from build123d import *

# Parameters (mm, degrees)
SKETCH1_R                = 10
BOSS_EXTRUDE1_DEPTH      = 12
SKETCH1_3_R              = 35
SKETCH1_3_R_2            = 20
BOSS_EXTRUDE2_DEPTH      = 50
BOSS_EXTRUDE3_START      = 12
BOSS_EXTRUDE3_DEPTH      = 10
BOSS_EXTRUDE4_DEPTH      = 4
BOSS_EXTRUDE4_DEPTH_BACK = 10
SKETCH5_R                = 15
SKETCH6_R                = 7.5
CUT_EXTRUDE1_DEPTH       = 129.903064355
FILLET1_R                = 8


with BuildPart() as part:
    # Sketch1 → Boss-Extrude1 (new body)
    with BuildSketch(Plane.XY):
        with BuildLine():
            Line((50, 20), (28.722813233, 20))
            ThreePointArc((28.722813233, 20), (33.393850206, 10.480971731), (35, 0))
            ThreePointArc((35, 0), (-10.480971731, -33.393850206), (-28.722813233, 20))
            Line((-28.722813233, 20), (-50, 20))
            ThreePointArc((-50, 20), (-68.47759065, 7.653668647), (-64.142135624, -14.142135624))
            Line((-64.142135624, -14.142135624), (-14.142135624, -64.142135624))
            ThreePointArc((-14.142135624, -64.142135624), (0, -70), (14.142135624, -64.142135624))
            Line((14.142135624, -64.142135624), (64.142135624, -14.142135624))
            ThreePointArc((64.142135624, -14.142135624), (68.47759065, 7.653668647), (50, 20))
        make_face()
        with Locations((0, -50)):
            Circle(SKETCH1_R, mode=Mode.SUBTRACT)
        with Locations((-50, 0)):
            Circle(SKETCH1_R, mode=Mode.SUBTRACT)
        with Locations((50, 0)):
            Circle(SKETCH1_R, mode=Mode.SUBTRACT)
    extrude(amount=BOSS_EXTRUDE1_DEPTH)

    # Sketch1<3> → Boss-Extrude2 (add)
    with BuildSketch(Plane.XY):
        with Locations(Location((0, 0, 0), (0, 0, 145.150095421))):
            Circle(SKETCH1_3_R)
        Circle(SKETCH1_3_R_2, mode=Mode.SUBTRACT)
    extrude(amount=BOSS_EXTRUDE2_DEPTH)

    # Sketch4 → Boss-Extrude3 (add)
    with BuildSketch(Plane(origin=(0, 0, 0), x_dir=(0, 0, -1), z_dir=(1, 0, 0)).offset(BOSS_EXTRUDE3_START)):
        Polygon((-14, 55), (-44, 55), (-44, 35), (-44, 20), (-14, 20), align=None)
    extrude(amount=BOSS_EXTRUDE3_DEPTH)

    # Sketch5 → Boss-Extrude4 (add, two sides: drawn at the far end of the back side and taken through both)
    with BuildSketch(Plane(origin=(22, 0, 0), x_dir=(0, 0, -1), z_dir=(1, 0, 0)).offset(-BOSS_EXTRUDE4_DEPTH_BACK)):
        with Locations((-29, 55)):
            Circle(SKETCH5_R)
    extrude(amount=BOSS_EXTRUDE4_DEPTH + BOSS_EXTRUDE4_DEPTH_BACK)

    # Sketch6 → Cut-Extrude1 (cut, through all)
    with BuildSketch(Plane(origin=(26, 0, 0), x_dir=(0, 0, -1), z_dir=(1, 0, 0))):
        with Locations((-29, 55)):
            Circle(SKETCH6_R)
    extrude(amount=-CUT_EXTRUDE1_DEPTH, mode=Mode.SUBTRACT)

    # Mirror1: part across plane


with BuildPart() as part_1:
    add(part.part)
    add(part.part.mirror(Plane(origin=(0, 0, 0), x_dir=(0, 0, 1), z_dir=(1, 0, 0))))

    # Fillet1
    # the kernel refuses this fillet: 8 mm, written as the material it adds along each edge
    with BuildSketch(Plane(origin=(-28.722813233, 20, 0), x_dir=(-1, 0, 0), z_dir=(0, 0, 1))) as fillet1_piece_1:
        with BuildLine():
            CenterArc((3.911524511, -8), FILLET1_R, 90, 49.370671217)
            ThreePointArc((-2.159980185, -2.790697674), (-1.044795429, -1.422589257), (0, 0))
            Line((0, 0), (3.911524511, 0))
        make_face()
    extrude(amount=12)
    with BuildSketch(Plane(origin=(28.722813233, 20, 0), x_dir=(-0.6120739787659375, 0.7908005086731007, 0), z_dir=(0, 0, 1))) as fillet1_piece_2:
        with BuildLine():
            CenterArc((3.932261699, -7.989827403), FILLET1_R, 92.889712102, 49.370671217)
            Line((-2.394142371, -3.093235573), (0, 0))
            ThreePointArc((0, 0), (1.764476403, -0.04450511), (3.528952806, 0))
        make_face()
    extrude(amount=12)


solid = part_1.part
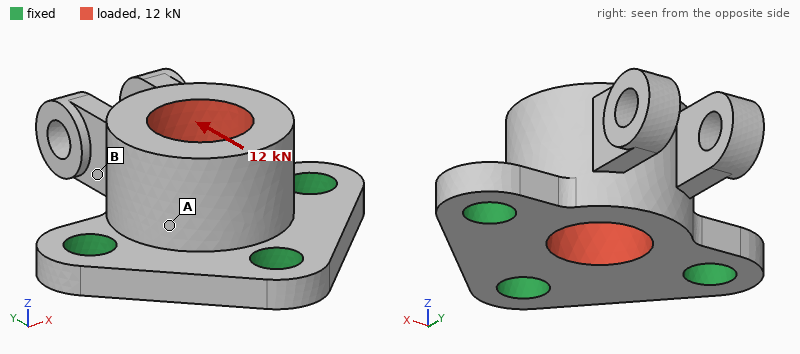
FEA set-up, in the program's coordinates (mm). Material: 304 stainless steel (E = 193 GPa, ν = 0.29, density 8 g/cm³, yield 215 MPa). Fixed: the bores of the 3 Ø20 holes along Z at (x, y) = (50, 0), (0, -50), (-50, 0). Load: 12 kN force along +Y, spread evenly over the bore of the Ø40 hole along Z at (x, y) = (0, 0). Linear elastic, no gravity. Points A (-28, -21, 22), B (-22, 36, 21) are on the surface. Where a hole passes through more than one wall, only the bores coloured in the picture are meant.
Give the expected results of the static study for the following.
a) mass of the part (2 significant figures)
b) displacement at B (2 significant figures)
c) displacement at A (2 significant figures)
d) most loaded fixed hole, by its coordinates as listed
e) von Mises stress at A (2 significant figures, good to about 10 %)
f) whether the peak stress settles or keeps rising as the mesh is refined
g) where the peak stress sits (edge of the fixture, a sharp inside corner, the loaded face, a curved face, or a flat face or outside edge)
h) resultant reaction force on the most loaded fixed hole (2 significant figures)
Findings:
1.6 kg
11 µm
4.7 µm
(0, -50)
11 MPa
keeps rising
edge of the fixture
7.1 kN
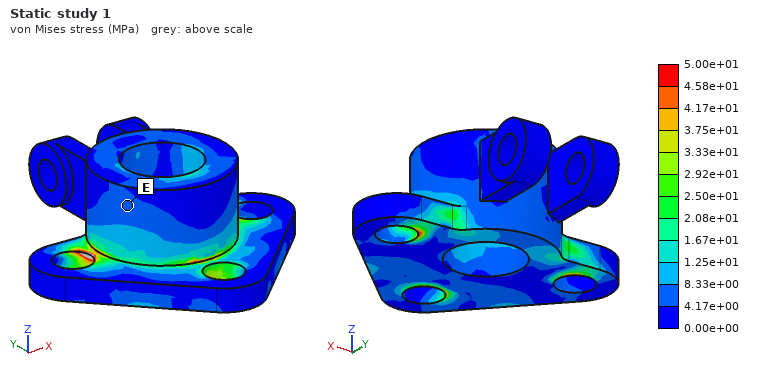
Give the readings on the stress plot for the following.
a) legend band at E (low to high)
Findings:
4.17e+00 to 8.33e+00 MPa
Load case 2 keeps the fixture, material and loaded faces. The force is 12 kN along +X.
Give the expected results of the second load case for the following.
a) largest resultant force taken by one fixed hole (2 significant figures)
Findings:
5.7 kN
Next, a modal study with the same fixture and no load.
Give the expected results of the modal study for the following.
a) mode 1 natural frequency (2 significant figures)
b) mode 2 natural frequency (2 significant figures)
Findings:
3300 Hz
4500 Hz
